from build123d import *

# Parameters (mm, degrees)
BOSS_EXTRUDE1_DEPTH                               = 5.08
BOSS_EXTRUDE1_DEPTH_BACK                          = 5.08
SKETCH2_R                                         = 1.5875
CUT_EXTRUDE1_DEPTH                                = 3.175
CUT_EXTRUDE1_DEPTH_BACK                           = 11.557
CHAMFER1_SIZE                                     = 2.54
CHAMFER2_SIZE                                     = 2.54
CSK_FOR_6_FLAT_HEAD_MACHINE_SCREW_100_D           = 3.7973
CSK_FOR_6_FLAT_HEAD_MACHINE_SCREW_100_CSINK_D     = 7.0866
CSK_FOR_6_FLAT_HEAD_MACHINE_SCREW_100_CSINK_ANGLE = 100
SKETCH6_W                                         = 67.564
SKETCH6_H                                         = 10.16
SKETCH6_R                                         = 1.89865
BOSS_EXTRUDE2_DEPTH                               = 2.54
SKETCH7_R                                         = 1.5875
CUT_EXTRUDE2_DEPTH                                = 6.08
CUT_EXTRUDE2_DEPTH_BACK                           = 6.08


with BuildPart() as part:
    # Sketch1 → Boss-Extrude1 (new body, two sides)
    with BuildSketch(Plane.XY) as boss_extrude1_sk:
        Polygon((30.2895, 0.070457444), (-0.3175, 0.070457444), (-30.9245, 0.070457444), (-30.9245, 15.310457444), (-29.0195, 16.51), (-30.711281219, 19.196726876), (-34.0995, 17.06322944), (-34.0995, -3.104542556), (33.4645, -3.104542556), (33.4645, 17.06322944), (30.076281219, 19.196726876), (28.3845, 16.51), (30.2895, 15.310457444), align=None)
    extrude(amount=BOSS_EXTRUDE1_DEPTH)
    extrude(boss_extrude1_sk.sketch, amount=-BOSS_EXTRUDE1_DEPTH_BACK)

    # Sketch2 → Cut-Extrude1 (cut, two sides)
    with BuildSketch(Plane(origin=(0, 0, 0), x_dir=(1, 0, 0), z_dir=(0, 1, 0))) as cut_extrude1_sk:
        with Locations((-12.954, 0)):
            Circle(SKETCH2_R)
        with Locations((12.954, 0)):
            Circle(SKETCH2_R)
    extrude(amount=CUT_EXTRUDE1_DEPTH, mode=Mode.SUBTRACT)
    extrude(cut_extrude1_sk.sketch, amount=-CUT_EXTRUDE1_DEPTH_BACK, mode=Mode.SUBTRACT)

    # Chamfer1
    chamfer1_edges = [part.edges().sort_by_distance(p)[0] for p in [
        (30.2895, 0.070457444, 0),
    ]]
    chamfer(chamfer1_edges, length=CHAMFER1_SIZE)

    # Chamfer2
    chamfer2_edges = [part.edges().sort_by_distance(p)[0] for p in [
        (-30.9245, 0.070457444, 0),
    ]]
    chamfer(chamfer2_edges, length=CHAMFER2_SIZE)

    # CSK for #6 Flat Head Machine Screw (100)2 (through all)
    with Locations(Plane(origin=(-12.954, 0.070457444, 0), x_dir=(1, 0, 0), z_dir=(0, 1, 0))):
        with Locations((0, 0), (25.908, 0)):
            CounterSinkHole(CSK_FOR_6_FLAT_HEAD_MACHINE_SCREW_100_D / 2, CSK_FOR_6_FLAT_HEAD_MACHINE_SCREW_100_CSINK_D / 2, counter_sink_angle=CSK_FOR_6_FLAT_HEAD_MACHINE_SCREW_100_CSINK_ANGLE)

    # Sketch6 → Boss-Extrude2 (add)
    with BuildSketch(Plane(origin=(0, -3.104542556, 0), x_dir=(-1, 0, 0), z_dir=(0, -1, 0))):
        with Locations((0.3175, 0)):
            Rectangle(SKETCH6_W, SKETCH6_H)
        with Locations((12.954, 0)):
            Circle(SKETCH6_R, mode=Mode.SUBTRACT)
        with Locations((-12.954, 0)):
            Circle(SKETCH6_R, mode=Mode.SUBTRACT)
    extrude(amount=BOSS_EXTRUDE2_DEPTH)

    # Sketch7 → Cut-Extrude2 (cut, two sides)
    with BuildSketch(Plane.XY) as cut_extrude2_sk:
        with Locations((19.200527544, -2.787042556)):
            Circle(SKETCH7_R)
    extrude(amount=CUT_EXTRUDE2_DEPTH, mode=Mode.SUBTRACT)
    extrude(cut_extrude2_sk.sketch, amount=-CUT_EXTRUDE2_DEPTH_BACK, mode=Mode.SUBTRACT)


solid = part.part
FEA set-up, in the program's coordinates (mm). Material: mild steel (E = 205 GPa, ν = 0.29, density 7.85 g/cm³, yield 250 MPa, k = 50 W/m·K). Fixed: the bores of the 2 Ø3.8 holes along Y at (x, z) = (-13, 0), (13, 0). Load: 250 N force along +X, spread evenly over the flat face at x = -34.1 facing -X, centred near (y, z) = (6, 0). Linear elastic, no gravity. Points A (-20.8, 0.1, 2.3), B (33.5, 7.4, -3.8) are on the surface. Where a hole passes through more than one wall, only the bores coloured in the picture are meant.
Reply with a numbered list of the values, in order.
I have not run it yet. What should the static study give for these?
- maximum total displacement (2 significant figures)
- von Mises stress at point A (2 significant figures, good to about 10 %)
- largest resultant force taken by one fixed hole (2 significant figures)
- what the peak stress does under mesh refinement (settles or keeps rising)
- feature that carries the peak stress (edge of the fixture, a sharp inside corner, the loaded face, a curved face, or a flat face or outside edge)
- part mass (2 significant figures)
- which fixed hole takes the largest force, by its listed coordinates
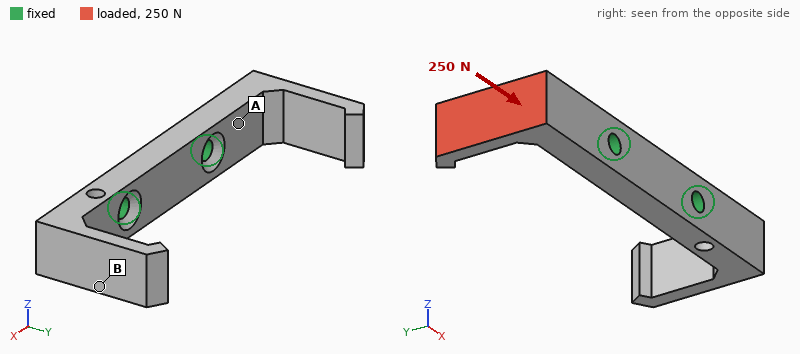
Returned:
1. 49 µm
2. 42 MPa
3. 220 N
4. keeps rising
5. edge of the fixture
6. 39 g
7. (-13, 0)
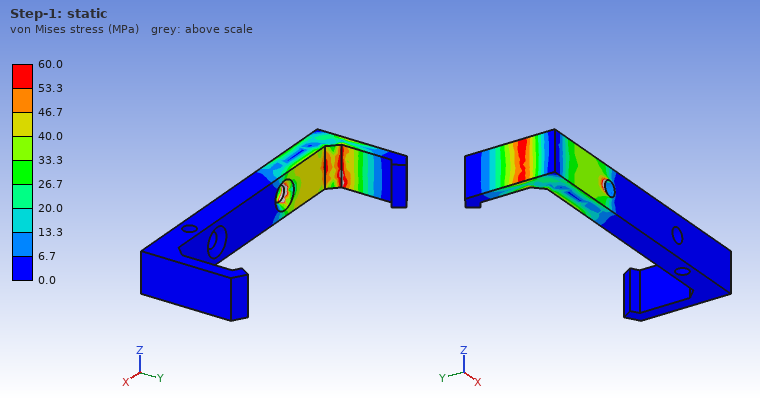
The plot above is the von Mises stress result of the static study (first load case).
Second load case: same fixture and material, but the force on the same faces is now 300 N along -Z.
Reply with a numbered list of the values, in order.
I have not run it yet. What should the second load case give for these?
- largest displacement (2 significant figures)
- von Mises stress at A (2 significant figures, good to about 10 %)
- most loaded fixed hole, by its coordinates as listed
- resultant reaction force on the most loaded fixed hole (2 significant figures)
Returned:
1. 45 µm
2. 61 MPa
3. (-13, 0)
4. 400 N
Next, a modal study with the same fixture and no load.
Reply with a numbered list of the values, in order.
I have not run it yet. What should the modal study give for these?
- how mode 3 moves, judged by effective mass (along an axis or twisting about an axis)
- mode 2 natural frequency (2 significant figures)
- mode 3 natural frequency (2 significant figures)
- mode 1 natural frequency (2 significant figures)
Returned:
1. along Z
2. 4300 Hz
3. 5300 Hz
4. 4300 Hz
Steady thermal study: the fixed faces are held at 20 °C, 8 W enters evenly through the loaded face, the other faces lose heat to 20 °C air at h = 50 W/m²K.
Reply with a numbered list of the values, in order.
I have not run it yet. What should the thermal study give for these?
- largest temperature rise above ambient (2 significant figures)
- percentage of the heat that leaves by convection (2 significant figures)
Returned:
1. 66 K
2. 22 %
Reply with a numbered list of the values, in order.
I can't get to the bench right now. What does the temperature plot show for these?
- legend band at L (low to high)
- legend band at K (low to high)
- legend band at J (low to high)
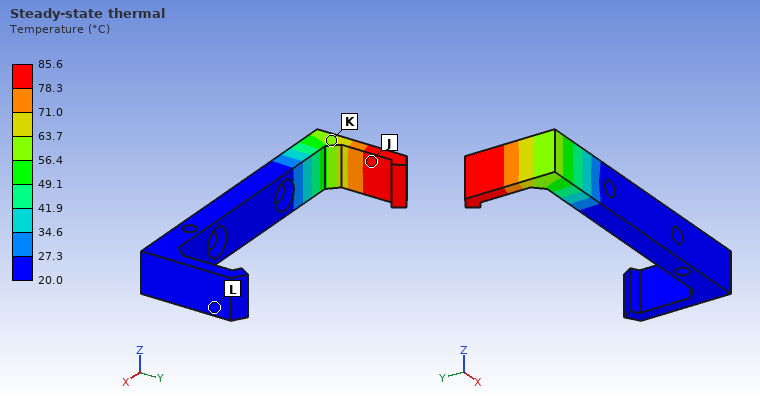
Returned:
1. 20.0 to 27.3 °C
2. 56.4 to 63.7 °C
3. 78.3 to 85.6 °C
